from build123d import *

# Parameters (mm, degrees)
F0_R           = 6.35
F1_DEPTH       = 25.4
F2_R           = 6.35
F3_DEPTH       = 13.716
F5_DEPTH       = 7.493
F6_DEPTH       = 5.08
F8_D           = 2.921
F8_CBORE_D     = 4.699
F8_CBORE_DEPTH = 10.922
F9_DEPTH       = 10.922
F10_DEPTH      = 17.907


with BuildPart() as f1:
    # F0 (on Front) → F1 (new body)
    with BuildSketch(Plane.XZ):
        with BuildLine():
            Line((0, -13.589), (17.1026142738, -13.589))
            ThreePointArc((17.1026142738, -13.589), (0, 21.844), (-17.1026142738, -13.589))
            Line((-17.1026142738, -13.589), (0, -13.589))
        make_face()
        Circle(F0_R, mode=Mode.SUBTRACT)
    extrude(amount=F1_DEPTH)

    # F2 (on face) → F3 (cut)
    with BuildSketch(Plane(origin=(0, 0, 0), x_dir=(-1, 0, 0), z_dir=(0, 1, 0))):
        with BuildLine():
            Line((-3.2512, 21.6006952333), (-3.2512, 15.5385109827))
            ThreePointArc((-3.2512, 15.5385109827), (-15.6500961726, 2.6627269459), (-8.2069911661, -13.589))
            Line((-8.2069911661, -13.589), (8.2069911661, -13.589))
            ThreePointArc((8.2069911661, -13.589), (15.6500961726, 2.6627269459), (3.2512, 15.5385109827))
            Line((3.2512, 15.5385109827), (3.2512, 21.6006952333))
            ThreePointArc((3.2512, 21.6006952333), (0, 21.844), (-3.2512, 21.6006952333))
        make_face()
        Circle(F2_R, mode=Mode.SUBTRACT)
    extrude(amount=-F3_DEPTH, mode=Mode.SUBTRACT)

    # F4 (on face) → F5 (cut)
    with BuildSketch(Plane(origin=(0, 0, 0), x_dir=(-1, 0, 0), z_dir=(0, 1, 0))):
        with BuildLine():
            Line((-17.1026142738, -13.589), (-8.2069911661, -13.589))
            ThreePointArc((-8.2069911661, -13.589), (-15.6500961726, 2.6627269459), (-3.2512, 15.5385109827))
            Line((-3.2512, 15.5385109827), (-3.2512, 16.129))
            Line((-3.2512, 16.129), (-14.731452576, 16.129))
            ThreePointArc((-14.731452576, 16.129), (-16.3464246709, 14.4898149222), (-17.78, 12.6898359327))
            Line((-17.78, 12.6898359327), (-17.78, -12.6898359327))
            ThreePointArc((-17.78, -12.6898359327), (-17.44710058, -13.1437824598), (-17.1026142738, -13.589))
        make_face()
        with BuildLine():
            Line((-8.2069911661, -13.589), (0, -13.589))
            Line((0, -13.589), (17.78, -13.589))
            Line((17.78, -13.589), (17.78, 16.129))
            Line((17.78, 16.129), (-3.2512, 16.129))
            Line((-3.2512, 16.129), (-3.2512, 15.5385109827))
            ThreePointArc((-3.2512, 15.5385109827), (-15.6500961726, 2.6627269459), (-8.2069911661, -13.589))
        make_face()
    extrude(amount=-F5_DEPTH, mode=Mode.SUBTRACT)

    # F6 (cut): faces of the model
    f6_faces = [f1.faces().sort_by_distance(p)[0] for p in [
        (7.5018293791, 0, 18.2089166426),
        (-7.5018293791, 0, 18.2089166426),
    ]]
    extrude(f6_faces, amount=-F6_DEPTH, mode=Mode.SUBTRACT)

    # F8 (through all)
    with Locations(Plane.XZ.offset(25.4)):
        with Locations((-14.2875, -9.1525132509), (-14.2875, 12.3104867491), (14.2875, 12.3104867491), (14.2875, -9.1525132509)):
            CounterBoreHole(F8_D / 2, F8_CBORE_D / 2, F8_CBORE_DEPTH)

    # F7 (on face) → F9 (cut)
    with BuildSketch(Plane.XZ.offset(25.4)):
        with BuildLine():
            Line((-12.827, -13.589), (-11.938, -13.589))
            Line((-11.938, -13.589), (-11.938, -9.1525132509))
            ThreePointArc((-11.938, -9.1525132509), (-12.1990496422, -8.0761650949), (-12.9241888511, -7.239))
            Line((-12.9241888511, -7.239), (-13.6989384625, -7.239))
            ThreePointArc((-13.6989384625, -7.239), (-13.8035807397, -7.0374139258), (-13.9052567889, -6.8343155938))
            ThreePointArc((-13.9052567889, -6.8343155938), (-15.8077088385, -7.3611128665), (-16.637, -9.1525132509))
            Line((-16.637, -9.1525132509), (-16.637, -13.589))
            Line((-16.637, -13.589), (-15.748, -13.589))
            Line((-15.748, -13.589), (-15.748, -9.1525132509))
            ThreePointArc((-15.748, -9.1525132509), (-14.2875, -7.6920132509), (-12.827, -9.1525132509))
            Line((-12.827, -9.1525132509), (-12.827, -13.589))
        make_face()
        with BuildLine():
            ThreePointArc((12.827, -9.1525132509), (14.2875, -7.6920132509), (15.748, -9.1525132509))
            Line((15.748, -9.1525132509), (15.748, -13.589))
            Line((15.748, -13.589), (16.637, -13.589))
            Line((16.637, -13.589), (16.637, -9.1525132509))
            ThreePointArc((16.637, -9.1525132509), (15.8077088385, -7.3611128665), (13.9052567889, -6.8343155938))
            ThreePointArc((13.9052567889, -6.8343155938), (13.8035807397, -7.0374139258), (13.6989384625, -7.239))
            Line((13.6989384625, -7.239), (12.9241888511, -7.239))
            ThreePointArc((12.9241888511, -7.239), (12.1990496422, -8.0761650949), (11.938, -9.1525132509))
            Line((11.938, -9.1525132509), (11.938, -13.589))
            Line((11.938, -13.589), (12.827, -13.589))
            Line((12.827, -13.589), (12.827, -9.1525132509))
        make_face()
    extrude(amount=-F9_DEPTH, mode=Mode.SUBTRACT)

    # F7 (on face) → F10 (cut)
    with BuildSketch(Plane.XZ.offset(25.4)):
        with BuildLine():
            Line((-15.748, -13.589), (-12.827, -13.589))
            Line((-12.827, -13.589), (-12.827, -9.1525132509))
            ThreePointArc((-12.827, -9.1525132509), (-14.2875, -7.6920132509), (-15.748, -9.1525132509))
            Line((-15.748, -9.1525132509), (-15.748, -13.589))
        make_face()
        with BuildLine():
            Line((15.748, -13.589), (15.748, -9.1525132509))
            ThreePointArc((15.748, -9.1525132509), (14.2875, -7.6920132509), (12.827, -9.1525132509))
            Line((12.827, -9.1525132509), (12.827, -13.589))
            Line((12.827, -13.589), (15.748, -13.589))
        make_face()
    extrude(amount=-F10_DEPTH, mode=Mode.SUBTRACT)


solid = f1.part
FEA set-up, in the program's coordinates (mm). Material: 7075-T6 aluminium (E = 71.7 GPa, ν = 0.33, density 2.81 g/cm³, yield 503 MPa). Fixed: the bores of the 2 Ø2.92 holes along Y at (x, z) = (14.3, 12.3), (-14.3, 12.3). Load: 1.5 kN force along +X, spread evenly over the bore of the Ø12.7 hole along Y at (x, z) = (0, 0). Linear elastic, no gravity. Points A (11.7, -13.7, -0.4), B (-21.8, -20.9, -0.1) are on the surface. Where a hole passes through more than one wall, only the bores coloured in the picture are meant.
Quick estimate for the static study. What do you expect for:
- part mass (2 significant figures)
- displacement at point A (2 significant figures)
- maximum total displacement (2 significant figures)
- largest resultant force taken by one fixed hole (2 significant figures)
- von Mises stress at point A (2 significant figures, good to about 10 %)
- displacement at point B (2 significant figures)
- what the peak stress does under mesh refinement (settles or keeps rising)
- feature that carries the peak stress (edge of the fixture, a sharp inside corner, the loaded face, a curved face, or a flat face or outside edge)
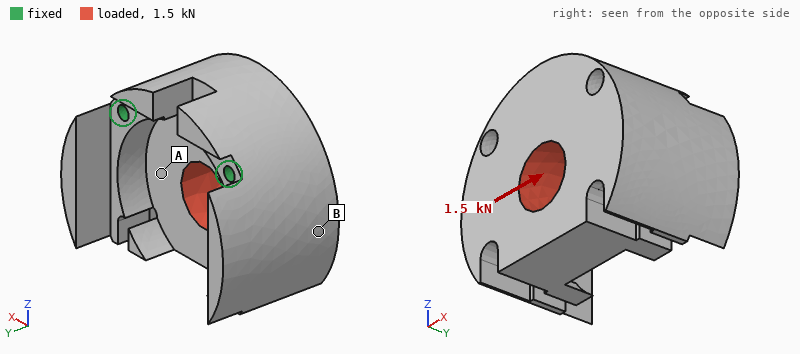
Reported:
47 g
7.5 µm
13 µm
1.0 kN
13 MPa
9.0 µm
keeps rising
edge of the fixture
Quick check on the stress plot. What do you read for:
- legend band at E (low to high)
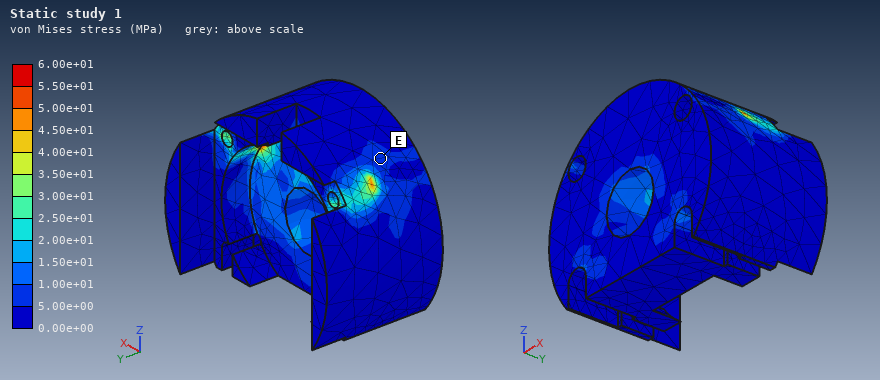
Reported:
5.00e+00 to 1.00e+01 MPa
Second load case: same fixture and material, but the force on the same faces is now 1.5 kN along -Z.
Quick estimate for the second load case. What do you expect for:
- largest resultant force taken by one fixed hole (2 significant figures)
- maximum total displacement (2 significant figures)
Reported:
750 N
34 µm
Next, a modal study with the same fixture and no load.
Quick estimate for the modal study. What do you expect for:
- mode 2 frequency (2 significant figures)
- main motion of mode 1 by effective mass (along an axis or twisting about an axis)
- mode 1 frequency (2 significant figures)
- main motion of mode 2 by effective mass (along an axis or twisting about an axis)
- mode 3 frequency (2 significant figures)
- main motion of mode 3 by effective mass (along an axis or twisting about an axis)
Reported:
9500 Hz
along Y
4900 Hz
along X
15 kHz
along X
